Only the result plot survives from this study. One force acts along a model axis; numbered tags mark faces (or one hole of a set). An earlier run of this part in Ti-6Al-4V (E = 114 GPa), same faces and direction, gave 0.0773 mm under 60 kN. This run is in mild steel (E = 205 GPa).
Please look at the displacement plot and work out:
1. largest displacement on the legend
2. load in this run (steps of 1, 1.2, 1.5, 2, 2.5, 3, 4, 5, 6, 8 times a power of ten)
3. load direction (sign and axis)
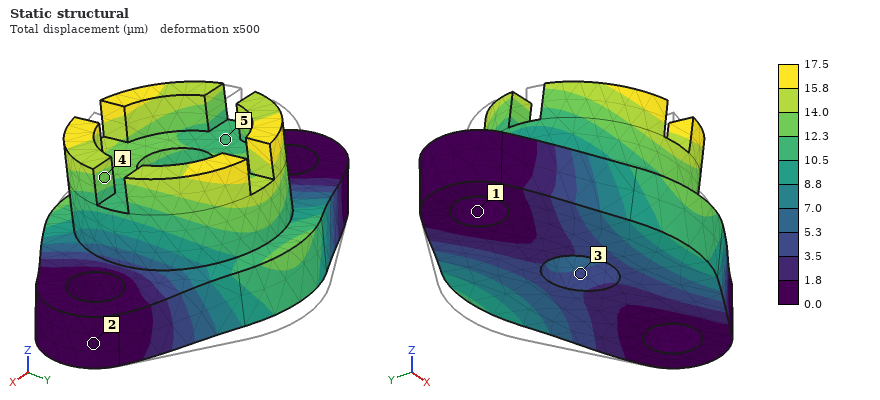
17.5 µm
25 kN
-Y
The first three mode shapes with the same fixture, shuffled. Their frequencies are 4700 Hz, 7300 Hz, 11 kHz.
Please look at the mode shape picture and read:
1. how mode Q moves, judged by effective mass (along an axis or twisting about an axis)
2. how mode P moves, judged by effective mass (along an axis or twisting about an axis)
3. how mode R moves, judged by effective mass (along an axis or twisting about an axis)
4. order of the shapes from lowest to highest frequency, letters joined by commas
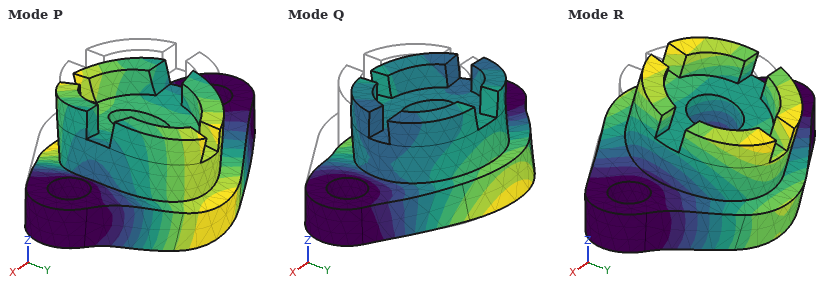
along Y
along Z
along Y
R, P, Q
